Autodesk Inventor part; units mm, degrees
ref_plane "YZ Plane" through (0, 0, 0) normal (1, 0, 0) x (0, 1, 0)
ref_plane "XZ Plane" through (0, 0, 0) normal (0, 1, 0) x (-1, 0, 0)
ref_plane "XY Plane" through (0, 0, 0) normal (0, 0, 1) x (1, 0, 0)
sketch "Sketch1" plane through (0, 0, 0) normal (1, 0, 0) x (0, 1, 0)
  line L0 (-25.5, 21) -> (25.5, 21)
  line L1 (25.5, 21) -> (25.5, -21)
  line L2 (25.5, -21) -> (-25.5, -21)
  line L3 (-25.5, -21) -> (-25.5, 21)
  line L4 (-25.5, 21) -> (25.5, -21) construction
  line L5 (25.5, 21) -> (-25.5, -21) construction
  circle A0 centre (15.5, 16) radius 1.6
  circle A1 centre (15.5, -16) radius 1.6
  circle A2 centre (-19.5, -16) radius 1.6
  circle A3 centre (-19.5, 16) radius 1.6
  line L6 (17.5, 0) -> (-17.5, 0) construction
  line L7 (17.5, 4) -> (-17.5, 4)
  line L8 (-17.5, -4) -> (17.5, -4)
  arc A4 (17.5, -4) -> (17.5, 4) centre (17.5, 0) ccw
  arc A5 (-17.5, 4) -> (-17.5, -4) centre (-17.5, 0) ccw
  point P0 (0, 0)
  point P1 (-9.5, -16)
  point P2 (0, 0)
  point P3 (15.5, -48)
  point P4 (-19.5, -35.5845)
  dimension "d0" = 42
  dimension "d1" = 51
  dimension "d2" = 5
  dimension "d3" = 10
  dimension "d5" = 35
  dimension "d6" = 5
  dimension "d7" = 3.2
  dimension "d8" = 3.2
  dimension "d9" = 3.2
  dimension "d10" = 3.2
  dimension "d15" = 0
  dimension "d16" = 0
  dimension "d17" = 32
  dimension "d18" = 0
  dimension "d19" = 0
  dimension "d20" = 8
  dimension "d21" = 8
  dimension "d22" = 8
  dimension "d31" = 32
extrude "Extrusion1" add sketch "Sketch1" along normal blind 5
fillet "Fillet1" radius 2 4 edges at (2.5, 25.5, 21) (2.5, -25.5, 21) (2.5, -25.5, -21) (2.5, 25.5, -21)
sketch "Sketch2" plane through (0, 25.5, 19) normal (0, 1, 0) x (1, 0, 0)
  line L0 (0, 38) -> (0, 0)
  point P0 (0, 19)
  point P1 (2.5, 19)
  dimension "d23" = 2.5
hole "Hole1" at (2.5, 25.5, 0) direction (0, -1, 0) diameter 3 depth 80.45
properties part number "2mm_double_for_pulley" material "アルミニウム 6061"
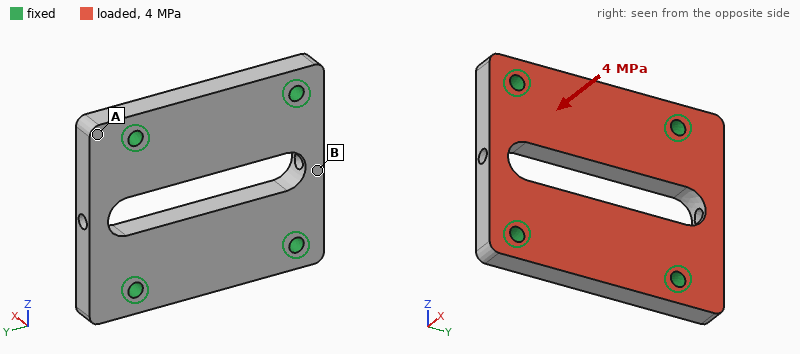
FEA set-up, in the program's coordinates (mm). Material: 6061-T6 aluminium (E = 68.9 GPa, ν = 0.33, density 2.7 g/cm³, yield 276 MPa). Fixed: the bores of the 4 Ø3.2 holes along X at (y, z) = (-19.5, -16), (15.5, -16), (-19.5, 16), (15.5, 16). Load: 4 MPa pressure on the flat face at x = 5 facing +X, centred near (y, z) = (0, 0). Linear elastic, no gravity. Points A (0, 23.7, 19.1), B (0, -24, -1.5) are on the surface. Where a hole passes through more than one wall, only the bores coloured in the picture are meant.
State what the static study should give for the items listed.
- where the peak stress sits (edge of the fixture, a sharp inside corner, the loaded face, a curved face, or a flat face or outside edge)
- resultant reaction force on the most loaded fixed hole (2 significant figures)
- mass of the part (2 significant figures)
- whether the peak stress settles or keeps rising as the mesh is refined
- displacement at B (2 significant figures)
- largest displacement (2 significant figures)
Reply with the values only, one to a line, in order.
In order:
edge of the fixture
1.9 kN
24 g
keeps rising
21 µm
58 µm
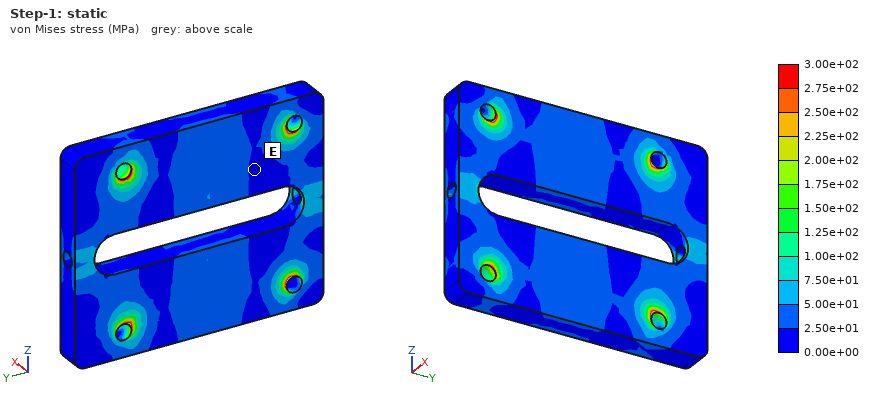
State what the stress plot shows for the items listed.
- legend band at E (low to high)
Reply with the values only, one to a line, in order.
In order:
0.00e+00 to 2.50e+01 MPa
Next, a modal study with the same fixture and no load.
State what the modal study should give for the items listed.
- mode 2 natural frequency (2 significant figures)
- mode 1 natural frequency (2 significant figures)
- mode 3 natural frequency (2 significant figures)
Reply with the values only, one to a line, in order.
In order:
15 kHz
15 kHz
20 kHz
